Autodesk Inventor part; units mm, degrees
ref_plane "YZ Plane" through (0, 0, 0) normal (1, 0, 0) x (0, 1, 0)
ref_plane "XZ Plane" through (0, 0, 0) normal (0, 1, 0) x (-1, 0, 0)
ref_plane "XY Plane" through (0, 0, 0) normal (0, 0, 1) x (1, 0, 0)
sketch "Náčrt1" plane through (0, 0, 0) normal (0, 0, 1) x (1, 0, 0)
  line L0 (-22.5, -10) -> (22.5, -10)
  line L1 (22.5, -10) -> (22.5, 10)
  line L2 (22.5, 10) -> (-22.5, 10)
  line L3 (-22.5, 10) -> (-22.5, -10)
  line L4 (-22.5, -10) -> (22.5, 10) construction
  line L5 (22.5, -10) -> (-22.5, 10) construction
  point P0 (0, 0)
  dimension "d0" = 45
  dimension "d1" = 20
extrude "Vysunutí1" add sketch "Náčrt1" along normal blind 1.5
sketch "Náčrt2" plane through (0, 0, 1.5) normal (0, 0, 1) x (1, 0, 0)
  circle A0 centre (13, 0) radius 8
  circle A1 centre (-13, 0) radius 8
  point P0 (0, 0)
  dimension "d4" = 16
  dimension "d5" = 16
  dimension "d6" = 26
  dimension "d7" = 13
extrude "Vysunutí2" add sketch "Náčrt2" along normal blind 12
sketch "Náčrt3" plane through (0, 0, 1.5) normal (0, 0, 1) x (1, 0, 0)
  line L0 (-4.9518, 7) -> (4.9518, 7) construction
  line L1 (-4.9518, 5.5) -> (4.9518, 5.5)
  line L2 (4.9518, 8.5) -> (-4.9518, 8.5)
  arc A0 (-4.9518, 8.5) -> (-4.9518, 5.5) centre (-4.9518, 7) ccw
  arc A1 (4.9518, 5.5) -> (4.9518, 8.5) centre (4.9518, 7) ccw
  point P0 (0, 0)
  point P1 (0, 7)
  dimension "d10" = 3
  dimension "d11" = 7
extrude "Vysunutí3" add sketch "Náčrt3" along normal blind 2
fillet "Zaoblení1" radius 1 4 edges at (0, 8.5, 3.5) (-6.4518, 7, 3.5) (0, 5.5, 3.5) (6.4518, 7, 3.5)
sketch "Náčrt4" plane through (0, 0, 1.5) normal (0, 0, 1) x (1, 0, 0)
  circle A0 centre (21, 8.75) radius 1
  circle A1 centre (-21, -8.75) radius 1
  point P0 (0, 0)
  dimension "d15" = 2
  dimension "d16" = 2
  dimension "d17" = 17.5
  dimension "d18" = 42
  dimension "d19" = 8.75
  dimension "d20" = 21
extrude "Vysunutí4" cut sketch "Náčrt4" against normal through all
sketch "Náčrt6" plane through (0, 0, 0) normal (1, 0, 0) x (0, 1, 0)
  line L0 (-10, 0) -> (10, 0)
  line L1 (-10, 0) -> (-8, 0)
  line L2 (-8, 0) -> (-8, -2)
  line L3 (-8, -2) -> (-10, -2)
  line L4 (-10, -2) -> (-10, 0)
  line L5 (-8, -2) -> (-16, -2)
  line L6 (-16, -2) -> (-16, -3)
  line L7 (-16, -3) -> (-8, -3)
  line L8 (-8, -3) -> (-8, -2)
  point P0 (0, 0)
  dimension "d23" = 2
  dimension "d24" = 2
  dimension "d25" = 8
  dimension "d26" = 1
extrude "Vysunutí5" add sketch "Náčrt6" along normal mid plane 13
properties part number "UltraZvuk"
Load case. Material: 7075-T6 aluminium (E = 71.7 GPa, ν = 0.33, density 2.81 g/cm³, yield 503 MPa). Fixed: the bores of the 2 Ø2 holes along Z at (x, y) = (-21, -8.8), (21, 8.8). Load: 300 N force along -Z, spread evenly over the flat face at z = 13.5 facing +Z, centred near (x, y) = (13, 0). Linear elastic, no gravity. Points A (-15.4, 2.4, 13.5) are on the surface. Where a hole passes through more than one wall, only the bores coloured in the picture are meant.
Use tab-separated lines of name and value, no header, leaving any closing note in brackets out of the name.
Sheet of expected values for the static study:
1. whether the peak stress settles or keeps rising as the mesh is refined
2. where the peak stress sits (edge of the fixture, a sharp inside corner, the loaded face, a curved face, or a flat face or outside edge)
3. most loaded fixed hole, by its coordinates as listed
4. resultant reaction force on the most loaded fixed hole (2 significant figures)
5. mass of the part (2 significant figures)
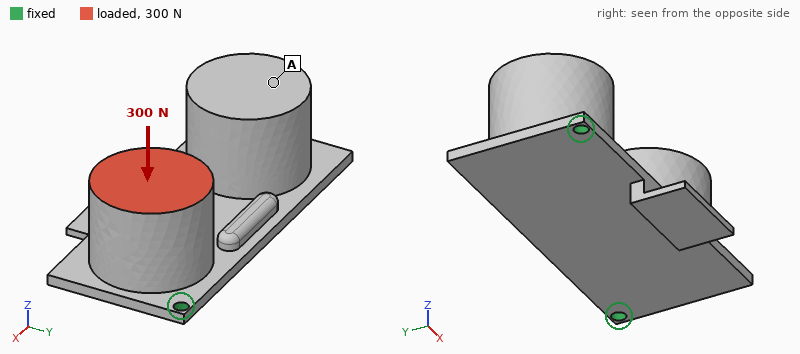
whether the peak stress settles or keeps rising as the mesh is refined	keeps rising
where the peak stress sits	edge of the fixture
most loaded fixed hole, by its coordinates as listed	(21, 8.8)
resultant reaction force on the most loaded fixed hole	240 N
mass of the part	18 g
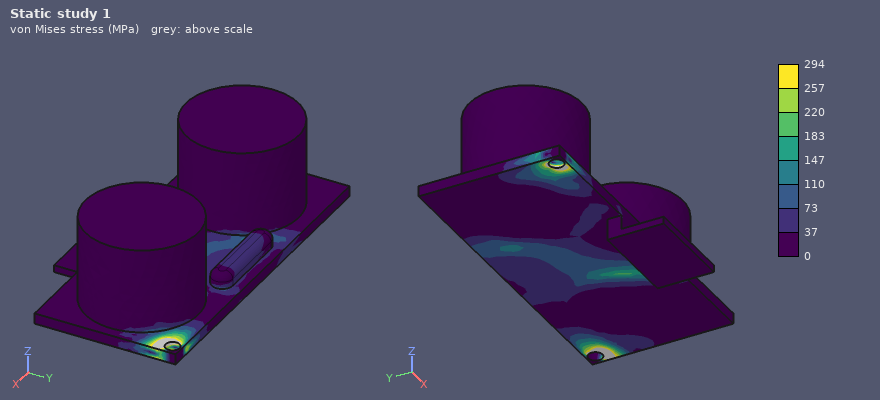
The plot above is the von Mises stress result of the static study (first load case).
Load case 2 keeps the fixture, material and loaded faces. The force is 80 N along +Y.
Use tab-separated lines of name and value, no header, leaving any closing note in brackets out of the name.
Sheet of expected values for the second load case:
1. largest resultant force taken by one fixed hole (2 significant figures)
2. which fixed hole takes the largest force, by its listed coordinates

largest resultant force taken by one fixed hole	67 N
which fixed hole takes the largest force, by its listed coordinates	(21, 8.8)
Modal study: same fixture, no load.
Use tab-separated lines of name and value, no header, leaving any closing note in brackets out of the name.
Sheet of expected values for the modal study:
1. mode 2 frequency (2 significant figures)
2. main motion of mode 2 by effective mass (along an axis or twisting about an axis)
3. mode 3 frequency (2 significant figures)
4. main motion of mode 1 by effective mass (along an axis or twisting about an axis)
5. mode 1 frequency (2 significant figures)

mode 2 frequency	1800 Hz
main motion of mode 2 by effective mass	along Z
mode 3 frequency	3100 Hz
main motion of mode 1 by effective mass	along Y
mode 1 frequency	1400 Hz
